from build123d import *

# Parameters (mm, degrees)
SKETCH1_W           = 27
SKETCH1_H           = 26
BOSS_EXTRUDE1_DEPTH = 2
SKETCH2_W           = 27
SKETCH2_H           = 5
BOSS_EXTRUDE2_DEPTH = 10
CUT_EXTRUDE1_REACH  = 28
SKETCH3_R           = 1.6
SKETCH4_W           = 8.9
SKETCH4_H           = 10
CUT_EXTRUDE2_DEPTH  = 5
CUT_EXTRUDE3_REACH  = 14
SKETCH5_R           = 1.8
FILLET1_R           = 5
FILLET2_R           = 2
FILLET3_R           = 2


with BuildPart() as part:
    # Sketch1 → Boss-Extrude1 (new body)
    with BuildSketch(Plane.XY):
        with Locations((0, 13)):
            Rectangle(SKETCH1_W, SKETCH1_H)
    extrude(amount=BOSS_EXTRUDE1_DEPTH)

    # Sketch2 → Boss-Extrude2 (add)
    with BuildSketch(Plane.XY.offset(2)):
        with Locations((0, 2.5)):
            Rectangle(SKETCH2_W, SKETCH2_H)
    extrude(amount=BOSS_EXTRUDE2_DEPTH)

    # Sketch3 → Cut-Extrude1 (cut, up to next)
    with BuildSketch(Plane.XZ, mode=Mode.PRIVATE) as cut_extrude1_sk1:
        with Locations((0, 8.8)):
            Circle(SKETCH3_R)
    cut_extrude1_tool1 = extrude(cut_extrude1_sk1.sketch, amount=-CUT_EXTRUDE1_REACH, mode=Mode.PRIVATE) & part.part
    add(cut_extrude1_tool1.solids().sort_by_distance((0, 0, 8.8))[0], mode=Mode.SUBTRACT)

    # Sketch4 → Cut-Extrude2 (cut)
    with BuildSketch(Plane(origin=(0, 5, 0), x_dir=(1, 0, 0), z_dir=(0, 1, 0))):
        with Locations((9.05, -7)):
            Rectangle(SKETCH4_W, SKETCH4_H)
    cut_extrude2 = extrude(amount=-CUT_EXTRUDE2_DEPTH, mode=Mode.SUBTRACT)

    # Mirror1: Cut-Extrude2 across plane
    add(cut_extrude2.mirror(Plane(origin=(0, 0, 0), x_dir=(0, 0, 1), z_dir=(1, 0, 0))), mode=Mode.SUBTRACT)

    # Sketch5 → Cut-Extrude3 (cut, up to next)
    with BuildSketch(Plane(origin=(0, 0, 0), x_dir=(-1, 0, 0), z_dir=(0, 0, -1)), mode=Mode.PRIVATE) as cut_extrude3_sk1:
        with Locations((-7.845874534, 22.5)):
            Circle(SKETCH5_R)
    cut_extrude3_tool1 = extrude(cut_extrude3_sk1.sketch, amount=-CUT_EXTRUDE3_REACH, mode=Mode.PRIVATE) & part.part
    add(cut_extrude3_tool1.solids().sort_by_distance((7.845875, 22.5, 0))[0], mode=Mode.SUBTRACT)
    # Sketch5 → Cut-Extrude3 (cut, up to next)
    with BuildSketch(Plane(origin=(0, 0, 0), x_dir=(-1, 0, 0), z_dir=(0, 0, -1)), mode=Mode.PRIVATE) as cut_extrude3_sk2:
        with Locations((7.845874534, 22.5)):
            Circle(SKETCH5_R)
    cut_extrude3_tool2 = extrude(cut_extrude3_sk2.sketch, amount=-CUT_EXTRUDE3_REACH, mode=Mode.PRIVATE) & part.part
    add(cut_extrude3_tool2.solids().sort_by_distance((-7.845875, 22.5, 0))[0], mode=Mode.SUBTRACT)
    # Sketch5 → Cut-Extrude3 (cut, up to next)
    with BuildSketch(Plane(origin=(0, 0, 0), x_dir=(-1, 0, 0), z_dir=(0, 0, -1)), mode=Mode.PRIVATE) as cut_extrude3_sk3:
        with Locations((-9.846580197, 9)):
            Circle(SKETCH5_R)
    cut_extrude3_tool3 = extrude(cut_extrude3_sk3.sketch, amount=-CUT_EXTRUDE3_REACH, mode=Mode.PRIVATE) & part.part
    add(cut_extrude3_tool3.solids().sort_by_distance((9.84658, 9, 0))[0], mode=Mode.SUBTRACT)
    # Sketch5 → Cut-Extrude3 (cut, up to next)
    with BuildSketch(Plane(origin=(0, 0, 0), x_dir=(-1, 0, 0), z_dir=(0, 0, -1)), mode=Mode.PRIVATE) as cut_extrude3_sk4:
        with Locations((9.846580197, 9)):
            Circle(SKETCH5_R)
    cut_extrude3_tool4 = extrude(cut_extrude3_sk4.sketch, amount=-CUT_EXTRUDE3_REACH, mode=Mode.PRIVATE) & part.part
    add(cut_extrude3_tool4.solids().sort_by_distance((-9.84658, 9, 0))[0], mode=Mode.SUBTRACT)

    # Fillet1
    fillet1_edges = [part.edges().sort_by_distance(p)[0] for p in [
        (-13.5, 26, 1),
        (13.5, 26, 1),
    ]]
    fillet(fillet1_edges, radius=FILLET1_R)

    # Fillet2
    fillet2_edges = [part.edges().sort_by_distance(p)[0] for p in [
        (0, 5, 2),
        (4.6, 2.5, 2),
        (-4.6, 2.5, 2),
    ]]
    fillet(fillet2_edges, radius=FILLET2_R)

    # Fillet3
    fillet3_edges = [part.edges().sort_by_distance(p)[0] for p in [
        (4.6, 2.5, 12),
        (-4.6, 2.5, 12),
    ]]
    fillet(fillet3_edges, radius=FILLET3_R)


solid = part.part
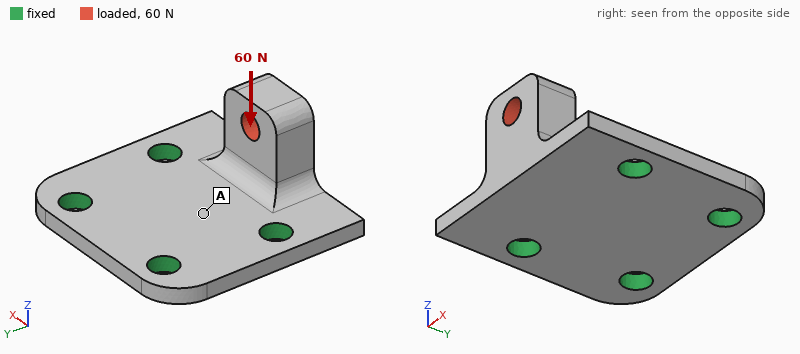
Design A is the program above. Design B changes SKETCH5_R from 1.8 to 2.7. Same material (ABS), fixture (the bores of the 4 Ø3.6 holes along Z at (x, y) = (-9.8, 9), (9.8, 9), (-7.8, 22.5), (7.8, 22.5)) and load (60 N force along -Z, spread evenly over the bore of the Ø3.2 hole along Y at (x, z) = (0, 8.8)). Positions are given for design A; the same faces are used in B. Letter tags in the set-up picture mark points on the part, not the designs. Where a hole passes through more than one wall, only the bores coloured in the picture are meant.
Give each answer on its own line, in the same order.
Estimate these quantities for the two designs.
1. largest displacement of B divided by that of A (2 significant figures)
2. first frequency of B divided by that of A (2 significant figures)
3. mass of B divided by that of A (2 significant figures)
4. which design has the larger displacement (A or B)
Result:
0.72
1.2
0.94
A
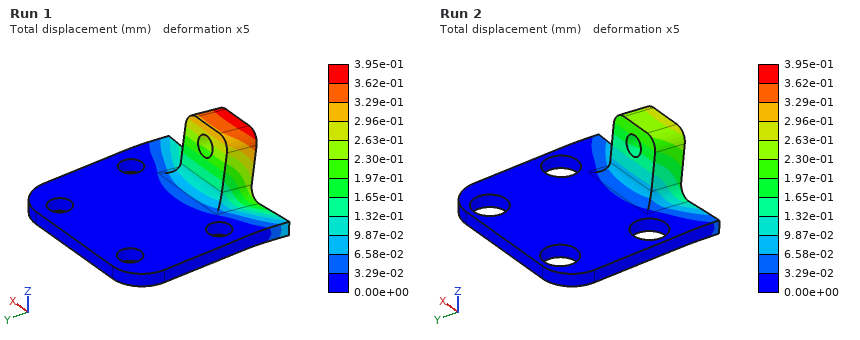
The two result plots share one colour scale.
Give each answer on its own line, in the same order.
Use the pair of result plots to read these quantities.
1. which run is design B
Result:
Run 2
